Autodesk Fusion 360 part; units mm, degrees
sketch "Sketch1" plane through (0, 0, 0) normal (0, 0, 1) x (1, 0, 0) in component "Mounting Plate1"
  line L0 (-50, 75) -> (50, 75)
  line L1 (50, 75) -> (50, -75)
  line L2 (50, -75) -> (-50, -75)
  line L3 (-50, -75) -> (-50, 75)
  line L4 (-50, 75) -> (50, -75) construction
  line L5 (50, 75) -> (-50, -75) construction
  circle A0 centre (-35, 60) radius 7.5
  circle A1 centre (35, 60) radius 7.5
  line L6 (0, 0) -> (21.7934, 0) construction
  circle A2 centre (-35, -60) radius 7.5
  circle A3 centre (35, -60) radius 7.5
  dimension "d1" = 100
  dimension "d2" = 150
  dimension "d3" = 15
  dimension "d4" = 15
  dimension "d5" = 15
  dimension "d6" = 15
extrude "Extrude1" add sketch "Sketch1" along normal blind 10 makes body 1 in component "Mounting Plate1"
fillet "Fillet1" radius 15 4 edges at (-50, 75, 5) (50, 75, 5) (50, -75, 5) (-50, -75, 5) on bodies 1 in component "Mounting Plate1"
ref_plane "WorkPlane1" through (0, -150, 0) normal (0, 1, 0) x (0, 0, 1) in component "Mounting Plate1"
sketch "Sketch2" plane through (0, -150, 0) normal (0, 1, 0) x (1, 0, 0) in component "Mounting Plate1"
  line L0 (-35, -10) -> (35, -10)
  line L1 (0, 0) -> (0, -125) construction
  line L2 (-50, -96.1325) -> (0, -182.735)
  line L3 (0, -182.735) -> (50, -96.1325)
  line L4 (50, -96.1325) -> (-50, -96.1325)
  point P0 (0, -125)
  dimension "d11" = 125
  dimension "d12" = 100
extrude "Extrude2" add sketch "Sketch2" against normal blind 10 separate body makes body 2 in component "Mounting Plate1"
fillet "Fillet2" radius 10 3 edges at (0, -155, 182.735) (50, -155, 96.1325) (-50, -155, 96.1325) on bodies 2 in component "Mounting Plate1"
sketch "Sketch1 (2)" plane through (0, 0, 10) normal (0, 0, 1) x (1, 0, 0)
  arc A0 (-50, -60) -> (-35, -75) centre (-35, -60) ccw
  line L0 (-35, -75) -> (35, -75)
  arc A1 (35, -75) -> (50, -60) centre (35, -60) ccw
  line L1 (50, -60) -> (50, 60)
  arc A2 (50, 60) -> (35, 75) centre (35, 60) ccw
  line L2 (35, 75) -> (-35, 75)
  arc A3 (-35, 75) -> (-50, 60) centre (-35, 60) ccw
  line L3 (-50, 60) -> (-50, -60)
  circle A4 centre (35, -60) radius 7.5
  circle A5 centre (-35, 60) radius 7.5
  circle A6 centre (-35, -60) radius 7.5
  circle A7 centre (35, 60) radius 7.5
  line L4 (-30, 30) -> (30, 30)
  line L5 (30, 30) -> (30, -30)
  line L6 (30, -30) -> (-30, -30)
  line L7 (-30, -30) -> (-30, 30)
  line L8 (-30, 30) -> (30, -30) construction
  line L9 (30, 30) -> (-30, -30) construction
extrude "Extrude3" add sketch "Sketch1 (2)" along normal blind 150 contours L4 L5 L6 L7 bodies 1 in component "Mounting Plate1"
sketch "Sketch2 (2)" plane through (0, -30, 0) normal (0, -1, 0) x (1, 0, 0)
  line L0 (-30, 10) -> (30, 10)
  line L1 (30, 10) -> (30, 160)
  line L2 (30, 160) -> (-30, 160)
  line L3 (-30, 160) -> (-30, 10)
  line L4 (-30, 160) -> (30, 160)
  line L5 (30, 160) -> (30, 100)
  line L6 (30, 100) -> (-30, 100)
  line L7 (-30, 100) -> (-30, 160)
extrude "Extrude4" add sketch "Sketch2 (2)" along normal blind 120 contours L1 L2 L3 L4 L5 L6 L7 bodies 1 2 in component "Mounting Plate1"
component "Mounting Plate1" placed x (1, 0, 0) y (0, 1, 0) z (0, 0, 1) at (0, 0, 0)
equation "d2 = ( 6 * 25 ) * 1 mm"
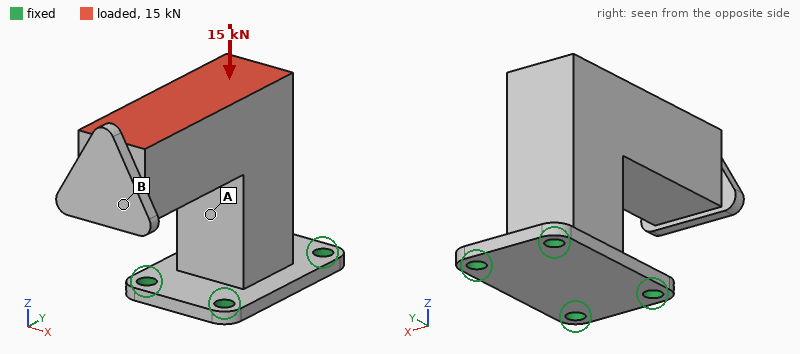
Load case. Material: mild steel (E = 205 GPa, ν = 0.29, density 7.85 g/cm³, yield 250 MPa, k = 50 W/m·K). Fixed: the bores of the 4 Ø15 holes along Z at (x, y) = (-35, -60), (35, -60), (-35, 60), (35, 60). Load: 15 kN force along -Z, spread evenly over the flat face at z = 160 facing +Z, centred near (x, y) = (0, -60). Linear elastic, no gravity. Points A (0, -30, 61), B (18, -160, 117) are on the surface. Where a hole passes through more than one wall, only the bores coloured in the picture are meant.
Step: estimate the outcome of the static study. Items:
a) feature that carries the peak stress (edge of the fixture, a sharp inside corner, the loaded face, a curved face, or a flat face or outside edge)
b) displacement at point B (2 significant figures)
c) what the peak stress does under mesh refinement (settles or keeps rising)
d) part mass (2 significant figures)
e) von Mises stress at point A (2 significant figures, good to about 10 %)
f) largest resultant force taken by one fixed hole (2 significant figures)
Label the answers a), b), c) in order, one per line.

a) edge of the fixture
b) 0.25 mm
c) keeps rising
d) 9.1 kg
e) 28 MPa
f) 9.0 kN
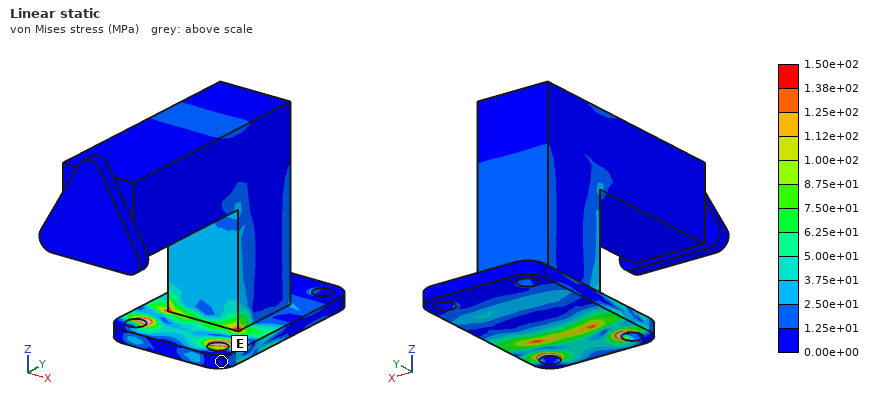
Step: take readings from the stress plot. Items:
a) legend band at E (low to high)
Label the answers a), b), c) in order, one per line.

a) 0.00e+00 to 1.25e+01 MPa
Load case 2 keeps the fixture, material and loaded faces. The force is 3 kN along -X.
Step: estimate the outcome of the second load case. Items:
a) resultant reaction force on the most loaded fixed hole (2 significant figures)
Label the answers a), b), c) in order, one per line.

a) 3.8 kN
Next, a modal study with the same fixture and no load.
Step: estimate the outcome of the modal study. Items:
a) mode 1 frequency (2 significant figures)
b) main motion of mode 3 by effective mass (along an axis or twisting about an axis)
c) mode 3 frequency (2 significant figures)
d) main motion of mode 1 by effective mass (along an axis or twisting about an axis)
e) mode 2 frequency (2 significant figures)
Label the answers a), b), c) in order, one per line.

a) 370 Hz
b) twisting about Z
c) 1200 Hz
d) along X
e) 420 Hz
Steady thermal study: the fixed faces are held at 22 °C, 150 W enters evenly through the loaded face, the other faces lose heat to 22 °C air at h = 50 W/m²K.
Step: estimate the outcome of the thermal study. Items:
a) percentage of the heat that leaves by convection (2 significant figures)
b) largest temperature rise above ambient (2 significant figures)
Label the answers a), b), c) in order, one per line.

a) 83 %
b) 57 K
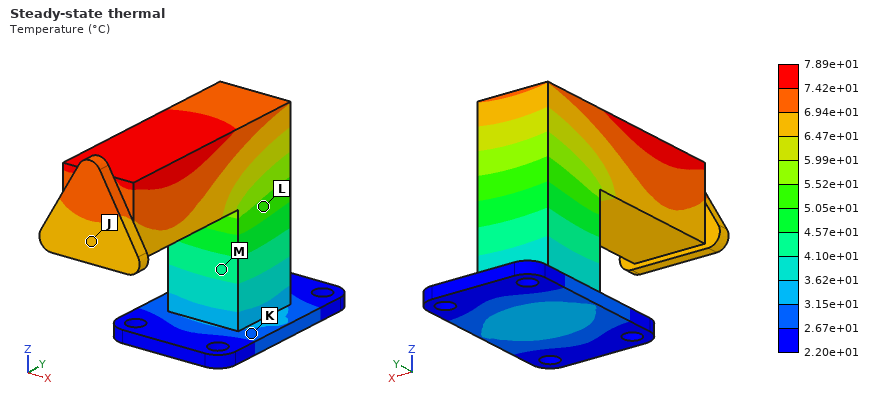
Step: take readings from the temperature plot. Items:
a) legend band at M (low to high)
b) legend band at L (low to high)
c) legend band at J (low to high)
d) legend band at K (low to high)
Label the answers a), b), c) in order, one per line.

a) 4.10e+01 to 4.57e+01 °C
b) 5.05e+01 to 5.52e+01 °C
c) 6.47e+01 to 6.94e+01 °C
d) 2.67e+01 to 3.15e+01 °C
